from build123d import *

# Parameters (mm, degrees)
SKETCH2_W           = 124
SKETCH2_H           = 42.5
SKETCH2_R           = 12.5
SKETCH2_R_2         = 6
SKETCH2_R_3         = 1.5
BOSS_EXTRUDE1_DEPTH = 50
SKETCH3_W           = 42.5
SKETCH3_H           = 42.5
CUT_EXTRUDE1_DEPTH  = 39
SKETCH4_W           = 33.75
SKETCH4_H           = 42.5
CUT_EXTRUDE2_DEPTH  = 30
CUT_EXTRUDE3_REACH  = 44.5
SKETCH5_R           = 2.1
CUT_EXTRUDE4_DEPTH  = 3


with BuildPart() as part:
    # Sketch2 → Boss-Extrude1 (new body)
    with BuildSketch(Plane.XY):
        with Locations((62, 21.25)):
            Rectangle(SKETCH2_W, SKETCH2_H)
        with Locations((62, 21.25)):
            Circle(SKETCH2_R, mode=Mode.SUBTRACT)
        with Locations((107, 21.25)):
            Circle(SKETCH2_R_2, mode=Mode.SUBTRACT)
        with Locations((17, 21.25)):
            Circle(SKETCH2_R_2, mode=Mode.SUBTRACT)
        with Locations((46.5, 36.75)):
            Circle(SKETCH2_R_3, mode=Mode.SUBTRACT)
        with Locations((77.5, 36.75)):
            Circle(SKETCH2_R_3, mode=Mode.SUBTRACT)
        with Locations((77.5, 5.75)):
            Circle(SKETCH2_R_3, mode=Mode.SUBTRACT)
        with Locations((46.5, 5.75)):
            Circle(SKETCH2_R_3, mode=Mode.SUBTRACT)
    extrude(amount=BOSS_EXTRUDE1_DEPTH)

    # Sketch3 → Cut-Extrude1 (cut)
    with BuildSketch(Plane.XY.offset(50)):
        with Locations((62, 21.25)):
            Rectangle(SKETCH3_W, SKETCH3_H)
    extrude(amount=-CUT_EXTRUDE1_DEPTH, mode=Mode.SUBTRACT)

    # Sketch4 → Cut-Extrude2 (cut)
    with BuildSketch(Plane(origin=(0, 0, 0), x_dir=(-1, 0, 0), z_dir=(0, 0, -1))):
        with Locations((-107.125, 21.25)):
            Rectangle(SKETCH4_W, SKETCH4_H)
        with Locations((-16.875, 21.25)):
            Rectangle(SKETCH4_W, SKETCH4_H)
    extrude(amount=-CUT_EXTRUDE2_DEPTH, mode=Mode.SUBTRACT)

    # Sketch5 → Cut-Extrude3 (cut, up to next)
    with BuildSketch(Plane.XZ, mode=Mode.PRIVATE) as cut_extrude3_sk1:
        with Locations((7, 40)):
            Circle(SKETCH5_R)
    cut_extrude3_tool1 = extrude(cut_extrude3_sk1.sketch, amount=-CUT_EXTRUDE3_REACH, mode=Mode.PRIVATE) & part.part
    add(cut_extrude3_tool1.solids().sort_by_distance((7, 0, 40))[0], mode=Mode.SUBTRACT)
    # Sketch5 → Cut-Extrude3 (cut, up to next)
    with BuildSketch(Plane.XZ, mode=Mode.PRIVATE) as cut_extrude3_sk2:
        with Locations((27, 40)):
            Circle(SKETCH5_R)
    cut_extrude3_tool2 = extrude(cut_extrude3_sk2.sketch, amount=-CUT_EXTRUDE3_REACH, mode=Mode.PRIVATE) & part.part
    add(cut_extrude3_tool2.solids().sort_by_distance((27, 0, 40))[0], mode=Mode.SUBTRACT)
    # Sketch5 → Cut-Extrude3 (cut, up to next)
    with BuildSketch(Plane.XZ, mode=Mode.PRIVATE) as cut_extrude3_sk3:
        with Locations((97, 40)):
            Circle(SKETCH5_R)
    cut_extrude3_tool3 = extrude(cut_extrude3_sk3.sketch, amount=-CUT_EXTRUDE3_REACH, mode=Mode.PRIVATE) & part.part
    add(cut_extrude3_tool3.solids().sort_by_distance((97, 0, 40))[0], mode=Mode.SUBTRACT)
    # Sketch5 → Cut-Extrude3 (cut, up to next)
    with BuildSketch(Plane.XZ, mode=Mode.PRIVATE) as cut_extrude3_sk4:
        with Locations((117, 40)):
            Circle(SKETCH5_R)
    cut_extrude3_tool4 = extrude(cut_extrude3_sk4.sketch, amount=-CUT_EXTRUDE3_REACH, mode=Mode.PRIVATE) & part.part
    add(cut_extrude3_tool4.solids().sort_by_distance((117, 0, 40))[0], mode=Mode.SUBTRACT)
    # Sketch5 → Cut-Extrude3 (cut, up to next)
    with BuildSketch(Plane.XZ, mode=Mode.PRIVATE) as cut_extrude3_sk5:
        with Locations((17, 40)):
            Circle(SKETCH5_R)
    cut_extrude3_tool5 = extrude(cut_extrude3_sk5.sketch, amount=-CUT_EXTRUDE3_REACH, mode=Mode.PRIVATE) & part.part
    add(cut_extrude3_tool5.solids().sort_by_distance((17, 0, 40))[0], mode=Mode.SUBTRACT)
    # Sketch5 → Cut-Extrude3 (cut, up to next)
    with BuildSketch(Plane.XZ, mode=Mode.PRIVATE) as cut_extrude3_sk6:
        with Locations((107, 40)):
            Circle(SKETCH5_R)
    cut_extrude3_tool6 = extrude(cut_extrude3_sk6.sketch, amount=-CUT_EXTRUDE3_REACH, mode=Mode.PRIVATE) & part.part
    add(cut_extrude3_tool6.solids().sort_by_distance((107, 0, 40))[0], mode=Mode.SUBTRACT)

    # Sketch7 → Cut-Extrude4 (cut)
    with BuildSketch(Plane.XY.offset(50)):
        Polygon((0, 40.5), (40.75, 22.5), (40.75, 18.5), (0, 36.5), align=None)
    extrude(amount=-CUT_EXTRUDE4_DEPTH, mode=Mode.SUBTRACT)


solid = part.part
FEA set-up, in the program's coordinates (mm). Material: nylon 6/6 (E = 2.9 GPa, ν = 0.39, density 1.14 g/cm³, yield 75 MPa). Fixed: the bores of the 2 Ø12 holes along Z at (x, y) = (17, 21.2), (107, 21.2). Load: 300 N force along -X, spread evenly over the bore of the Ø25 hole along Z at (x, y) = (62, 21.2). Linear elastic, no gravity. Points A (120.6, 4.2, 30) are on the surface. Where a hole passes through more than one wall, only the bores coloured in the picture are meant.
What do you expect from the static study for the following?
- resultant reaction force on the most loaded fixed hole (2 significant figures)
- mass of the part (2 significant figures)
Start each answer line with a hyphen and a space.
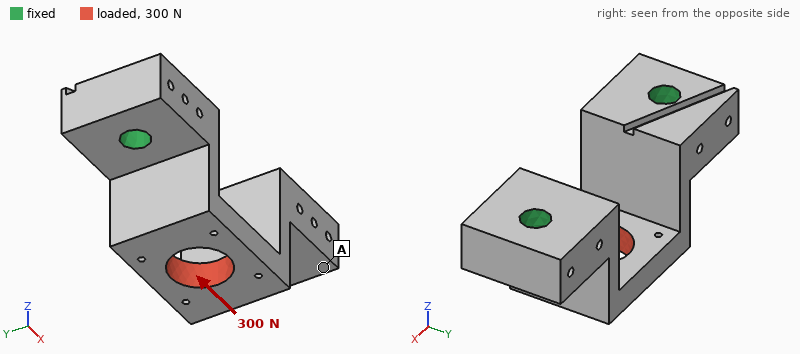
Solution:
- 170 N
- 110 g
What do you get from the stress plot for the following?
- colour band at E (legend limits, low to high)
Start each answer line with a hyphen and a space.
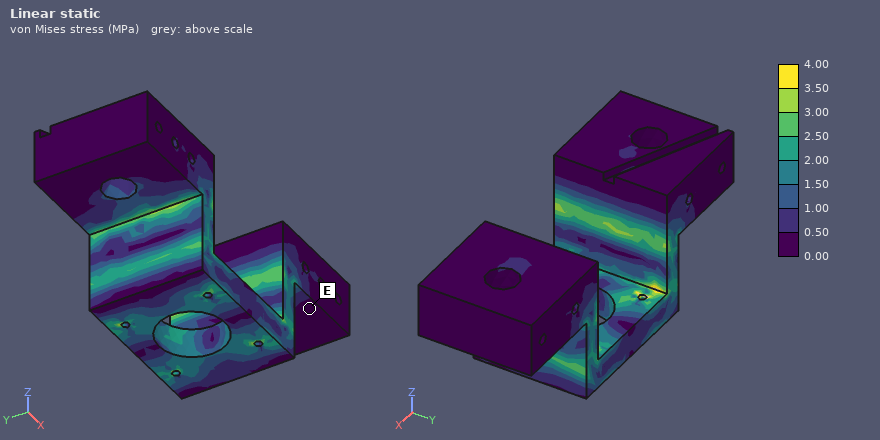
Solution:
- 0.00 to 0.50 MPa
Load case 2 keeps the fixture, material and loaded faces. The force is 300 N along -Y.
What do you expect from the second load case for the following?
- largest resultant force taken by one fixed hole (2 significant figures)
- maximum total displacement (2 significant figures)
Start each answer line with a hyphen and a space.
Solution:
- 150 N
- 0.10 mm
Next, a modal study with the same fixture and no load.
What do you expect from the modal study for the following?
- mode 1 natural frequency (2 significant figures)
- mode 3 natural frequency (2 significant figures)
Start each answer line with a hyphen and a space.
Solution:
- 1700 Hz
- 2300 Hz
